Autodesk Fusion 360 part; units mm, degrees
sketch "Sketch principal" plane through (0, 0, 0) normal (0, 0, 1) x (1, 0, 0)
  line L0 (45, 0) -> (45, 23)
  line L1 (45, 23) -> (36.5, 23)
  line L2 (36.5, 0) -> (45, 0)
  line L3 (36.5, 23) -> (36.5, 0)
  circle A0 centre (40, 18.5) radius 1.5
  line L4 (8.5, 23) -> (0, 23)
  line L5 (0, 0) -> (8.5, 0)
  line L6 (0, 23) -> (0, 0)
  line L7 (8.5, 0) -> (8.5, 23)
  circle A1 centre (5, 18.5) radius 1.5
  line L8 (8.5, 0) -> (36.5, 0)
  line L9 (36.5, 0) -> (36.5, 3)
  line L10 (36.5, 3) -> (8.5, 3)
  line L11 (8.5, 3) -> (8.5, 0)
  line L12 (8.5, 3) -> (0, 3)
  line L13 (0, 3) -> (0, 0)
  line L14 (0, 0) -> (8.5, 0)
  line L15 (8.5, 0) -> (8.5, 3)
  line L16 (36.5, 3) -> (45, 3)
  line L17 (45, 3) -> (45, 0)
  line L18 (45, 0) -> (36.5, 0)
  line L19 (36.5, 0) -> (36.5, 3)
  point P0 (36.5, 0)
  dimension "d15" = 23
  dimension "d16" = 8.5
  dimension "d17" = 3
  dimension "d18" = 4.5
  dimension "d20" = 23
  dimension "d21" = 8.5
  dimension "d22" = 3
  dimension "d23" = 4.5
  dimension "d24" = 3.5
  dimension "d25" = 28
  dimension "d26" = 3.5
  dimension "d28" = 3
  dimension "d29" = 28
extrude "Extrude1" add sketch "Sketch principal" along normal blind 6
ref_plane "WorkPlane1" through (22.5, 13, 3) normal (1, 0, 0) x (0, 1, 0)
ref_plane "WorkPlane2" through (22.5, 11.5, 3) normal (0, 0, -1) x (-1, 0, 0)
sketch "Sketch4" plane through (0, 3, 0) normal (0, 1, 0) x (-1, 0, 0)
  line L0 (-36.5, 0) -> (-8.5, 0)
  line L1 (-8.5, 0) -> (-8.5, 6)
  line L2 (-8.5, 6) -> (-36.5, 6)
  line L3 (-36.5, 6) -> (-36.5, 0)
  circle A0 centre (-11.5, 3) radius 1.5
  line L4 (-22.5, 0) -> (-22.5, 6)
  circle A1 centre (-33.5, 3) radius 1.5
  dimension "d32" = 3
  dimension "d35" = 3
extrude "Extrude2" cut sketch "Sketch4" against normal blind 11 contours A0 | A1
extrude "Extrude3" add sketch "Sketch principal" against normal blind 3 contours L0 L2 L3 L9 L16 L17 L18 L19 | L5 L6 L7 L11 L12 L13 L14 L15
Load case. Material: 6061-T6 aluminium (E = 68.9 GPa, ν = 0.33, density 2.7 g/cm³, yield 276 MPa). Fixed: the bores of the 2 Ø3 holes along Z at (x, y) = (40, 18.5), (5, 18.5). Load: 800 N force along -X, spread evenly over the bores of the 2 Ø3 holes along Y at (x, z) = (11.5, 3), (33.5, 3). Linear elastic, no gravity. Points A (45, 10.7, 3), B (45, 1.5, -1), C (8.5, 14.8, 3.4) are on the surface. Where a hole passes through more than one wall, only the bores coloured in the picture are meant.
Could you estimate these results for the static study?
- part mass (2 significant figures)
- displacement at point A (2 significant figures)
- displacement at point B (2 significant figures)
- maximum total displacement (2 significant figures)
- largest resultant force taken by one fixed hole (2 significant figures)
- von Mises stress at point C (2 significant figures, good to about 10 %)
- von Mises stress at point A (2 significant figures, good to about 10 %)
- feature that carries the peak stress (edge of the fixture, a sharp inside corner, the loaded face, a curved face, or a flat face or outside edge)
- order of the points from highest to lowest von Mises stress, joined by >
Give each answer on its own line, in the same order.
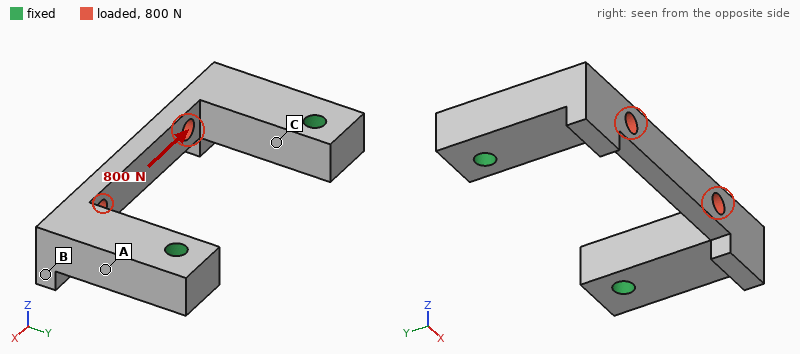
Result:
7.8 g
22 µm
51 µm
56 µm
400 N
68 MPa
43 MPa
edge of the fixture
C > A > B
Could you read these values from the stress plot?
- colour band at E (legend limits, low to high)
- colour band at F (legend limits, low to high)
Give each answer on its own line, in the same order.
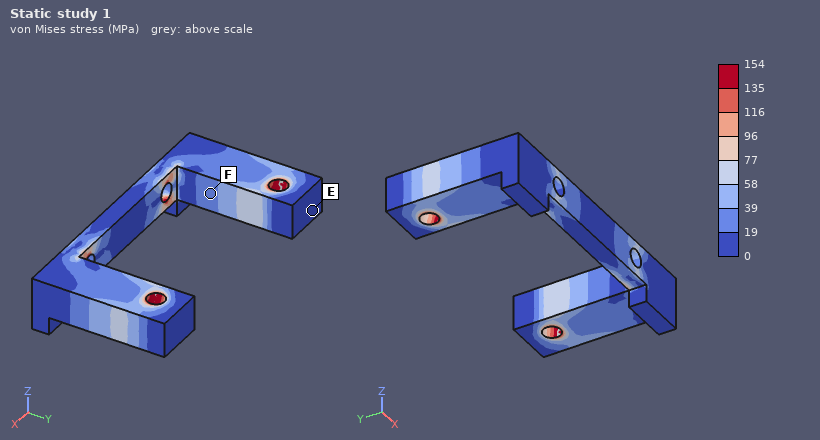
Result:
0 to 19 MPa
19 to 39 MPa
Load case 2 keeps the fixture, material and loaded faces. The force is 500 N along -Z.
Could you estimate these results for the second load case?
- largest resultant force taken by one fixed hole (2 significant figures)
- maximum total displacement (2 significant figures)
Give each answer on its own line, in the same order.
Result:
250 N
76 µm
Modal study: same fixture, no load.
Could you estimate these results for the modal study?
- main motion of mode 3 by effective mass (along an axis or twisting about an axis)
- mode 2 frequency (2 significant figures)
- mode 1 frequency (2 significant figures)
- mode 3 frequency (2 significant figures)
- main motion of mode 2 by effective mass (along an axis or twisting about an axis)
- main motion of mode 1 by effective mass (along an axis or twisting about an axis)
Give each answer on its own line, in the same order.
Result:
twisting about Y
11 kHz
8900 Hz
12 kHz
along X
along Z
